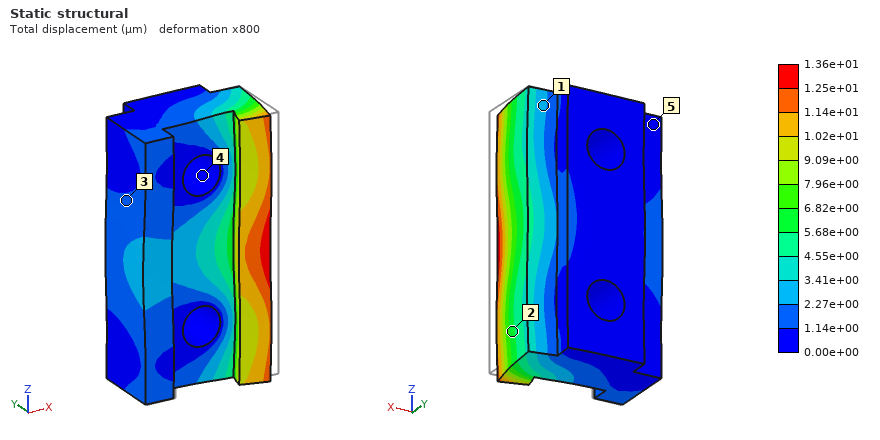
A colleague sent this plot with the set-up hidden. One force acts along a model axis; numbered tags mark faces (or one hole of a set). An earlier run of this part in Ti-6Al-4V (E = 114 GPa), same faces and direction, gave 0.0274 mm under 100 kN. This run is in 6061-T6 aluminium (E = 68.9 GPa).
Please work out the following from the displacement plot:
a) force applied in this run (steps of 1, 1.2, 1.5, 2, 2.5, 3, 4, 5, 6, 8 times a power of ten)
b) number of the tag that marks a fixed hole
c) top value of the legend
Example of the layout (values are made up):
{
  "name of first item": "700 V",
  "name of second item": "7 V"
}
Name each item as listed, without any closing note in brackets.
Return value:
{
  "force applied in this run": "30 kN",
  "number of the tag that marks a fixed hole": "4",
  "top value of the legend": "1.36e+01 µm"
}
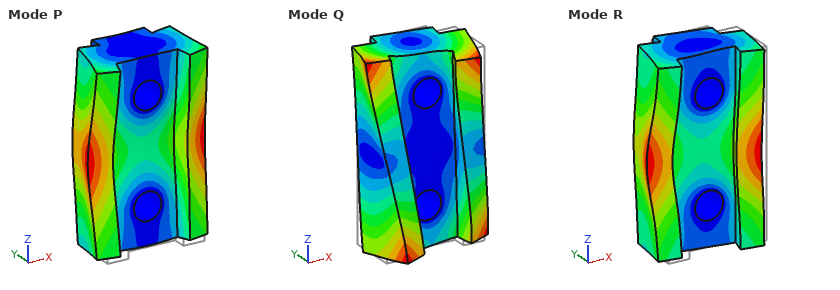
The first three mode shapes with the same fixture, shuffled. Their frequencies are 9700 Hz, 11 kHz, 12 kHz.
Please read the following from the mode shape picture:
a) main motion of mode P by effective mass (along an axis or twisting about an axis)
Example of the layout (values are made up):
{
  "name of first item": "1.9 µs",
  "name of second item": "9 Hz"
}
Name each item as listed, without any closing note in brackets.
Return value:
{
  "main motion of mode P by effective mass": "along Y"
}
